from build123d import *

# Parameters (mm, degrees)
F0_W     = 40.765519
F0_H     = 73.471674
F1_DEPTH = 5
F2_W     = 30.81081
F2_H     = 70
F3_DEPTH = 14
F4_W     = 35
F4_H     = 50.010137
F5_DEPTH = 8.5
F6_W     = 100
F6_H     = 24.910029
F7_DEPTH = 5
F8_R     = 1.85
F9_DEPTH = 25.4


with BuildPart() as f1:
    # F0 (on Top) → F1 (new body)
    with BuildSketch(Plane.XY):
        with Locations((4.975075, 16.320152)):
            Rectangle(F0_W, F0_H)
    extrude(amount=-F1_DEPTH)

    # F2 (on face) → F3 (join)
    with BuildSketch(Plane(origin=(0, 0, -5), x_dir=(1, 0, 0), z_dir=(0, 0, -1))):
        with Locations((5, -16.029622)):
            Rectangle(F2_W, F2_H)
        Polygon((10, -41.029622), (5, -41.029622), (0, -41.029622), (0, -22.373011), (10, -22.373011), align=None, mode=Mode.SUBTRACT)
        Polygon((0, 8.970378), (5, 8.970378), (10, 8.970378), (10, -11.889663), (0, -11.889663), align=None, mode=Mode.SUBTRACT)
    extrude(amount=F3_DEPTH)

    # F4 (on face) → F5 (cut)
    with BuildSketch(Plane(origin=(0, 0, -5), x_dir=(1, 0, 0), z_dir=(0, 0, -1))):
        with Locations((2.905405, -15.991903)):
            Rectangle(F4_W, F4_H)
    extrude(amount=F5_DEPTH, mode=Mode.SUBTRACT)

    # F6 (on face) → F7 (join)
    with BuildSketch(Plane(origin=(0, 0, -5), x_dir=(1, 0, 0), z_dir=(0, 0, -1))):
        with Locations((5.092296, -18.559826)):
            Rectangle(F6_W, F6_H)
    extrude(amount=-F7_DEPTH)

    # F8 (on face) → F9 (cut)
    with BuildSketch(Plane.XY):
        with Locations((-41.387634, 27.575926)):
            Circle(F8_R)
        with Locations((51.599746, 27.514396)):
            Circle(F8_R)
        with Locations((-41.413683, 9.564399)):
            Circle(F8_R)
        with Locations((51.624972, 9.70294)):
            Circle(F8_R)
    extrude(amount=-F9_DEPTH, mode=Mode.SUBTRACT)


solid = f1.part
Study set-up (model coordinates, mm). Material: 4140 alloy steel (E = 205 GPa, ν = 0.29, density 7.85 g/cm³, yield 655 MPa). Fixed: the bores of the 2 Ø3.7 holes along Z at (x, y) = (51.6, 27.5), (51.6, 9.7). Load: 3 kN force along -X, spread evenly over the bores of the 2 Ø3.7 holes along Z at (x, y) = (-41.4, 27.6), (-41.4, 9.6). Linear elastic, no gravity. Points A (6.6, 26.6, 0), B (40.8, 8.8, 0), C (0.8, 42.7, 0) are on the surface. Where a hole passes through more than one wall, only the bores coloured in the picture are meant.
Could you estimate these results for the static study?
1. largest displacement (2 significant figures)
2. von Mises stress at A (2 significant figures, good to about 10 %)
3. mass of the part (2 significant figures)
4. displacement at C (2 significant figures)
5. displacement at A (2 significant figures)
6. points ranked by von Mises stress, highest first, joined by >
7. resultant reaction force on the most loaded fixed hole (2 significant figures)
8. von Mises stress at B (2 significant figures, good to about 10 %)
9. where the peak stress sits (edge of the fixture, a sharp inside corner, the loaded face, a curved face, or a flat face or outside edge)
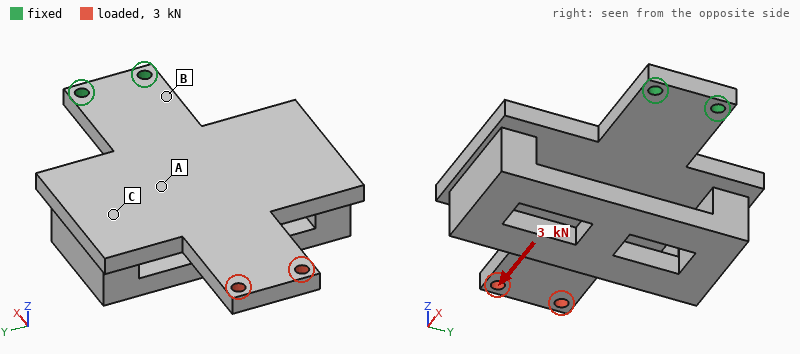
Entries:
12 µm
18 MPa
290 g
5.3 µm
5.1 µm
B > A > C
1.5 kN
27 MPa
the loaded face
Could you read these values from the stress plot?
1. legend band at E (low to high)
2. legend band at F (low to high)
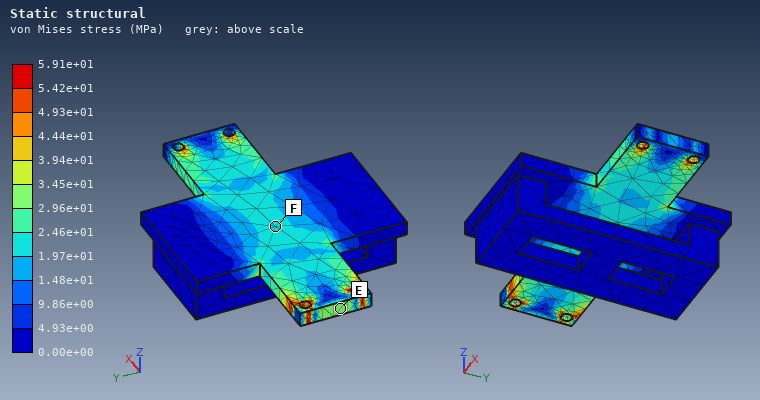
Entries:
2.96e+01 to 3.45e+01 MPa
1.97e+01 to 2.46e+01 MPa
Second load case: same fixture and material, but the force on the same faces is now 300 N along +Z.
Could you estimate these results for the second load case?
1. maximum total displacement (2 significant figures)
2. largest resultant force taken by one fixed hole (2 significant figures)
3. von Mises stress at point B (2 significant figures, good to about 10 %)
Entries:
1.3 mm
150 N
240 MPa
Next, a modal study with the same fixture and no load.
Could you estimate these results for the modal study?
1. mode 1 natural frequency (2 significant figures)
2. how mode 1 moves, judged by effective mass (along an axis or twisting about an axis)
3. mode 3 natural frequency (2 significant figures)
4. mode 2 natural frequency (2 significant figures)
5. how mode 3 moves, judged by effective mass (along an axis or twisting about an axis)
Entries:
320 Hz
along Z
1400 Hz
700 Hz
along Y
